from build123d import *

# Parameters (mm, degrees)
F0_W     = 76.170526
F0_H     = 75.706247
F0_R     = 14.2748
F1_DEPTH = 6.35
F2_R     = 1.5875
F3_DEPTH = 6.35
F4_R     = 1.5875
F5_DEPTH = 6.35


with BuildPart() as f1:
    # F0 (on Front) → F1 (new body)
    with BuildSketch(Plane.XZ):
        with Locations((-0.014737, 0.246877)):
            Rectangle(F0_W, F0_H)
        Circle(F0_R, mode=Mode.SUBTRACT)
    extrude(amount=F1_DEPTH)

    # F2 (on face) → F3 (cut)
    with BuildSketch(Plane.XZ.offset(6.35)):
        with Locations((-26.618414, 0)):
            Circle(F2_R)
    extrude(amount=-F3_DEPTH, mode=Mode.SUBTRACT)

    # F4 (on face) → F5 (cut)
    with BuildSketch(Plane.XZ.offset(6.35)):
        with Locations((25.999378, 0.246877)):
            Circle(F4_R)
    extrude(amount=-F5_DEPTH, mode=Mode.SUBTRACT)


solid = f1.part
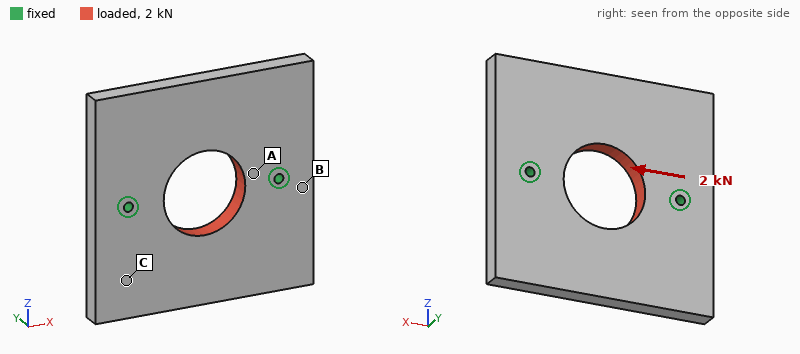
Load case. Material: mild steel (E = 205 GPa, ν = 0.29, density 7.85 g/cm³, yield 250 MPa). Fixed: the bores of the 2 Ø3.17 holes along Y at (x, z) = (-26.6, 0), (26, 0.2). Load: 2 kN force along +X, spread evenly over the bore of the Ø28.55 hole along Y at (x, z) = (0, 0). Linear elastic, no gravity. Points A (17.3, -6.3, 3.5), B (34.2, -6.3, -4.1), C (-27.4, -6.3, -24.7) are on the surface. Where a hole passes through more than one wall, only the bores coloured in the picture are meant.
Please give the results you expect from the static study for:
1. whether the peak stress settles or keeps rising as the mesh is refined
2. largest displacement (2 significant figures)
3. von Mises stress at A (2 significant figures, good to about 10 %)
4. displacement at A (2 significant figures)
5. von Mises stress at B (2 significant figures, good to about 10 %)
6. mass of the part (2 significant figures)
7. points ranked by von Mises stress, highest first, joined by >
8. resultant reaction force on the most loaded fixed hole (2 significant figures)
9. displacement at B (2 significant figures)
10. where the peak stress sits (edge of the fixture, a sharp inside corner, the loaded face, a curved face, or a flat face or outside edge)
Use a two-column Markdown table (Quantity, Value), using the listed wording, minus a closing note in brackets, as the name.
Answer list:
| Quantity | Value |
|---|---|
| whether the peak stress settles or keeps rising as the mesh is refined | keeps rising |
| largest displacement | 1.1 µm |
| von Mises stress at A | 7.4 MPa |
| displacement at A | 0.42 µm |
| von Mises stress at B | 4.1 MPa |
| mass of the part | 250 g |
| points ranked by von Mises stress, highest first, joined by > | A > B > C |
| resultant reaction force on the most loaded fixed hole | 1.0 kN |
| displacement at B | 0.28 µm |
| where the peak stress sits | edge of the fixture |
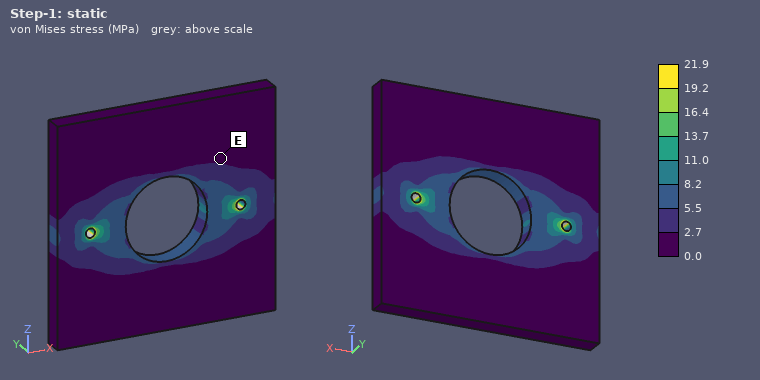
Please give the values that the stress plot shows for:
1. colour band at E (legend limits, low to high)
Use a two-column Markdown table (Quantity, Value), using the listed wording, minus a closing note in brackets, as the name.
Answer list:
| Quantity | Value |
|---|---|
| colour band at E | 0.0 to 2.7 MPa |
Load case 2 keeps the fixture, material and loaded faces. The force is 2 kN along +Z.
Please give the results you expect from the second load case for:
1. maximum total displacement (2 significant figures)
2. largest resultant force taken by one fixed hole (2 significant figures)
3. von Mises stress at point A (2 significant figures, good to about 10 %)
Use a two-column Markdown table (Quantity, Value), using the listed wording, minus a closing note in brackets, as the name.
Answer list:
| Quantity | Value |
|---|---|
| maximum total displacement | 1.1 µm |
| largest resultant force taken by one fixed hole | 1.0 kN |
| von Mises stress at point A | 6.6 MPa |
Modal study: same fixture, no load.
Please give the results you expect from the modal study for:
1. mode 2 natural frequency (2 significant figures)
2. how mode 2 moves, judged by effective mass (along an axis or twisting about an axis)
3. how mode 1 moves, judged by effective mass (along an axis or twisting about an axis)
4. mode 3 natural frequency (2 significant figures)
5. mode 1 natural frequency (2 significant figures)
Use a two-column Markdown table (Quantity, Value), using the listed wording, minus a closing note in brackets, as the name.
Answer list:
| Quantity | Value |
|---|---|
| mode 2 natural frequency | 3000 Hz |
| how mode 2 moves, judged by effective mass | along Y |
| how mode 1 moves, judged by effective mass | twisting about X |
| mode 3 natural frequency | 4500 Hz |
| mode 1 natural frequency | 2300 Hz |
